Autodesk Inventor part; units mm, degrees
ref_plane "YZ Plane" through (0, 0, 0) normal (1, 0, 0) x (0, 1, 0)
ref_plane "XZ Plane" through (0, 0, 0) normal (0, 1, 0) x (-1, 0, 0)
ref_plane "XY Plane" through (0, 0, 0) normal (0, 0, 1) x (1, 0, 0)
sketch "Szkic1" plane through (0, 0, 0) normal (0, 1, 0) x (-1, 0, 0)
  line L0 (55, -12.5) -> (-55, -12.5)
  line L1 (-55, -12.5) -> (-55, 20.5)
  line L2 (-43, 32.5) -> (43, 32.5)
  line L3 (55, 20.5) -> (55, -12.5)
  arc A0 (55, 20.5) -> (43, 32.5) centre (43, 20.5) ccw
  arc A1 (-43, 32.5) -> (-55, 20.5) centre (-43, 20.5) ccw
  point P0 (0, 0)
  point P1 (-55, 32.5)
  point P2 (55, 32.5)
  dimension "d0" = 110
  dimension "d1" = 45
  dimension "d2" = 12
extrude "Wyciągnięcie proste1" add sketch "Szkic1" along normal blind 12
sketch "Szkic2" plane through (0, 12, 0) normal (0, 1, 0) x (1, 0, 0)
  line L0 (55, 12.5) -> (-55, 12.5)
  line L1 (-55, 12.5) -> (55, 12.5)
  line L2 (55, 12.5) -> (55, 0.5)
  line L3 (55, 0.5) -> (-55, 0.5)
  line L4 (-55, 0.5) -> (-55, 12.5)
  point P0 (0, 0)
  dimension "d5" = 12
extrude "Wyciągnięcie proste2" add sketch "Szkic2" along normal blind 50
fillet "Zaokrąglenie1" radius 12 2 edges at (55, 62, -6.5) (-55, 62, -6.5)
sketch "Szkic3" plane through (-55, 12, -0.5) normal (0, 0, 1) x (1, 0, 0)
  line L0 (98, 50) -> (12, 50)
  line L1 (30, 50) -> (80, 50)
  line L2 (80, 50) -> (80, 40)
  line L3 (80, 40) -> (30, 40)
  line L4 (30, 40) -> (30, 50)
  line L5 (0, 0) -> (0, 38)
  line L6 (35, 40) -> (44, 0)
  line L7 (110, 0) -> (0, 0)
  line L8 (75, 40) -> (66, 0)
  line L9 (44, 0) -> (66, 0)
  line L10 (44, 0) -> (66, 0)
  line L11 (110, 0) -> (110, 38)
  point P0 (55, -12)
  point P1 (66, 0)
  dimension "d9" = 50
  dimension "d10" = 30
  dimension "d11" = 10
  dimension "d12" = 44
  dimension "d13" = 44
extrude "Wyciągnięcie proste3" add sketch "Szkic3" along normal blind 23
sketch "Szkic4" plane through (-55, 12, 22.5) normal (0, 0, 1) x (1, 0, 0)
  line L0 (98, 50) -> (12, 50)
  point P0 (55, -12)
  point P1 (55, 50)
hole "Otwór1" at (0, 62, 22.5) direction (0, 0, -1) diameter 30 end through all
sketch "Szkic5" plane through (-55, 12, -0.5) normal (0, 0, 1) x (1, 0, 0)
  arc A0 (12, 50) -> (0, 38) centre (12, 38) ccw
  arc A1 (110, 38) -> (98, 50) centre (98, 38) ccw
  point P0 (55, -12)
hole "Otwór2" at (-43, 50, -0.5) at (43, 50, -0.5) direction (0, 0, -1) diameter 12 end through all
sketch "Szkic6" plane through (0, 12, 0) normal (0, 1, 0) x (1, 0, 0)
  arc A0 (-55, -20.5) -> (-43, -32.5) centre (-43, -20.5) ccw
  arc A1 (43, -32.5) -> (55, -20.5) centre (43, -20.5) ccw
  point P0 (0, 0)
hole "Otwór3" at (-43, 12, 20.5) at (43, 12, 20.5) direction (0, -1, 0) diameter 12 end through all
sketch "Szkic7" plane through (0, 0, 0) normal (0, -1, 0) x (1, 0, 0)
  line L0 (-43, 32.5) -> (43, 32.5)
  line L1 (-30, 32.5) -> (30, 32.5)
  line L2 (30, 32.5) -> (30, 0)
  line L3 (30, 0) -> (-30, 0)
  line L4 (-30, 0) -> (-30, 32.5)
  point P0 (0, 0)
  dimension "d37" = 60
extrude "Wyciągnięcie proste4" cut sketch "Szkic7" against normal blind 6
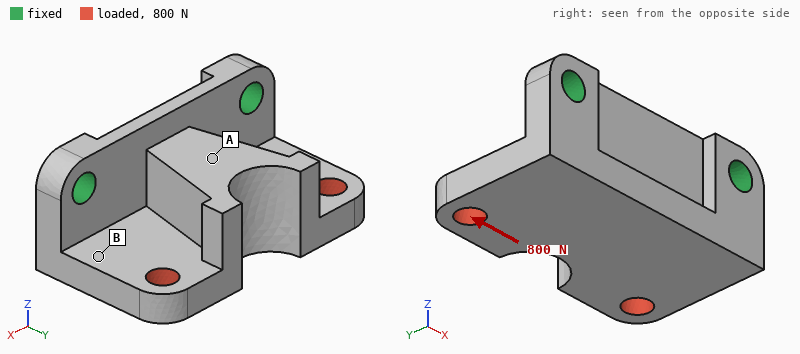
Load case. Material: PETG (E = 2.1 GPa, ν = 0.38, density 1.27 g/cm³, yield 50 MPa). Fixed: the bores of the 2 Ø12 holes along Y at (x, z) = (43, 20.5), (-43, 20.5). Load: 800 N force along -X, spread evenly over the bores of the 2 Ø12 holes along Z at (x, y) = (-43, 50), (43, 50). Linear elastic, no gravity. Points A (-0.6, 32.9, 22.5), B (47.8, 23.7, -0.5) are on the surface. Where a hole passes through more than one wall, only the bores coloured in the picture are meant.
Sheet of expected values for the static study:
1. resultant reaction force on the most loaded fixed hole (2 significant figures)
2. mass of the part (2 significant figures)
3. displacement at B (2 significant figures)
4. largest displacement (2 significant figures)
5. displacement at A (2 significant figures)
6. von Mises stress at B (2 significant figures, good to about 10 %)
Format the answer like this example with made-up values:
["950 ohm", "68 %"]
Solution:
["610 N", "170 g", "0.15 mm", "0.27 mm", "0.11 mm", "2.8 MPa"]
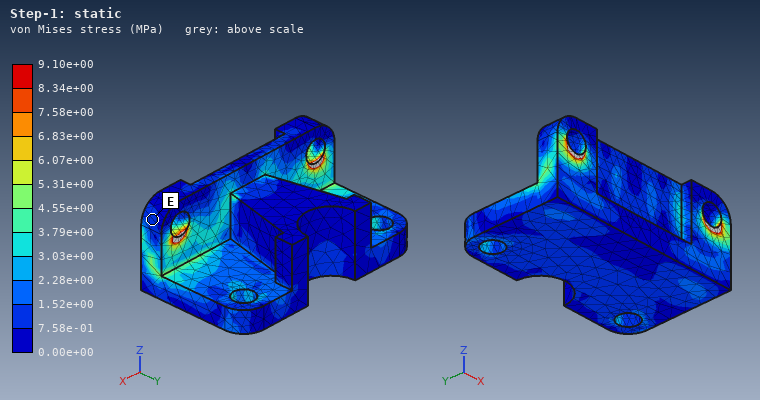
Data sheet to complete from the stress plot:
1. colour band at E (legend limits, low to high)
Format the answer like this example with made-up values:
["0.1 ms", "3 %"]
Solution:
["7.58e-01 to 1.52e+00 MPa"]
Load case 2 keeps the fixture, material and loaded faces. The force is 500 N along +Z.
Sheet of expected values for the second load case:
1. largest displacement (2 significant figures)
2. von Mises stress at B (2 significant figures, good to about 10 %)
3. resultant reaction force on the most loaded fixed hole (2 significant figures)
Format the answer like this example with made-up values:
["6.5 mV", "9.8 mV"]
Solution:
["1.5 mm", "3.5 MPa", "290 N"]
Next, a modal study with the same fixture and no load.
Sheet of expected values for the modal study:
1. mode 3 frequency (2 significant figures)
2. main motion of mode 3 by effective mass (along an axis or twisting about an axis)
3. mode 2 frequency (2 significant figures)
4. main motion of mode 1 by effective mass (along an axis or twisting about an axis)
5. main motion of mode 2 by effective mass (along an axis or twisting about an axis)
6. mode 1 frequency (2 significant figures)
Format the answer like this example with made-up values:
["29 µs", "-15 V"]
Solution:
["1100 Hz", "along Y", "1000 Hz", "along Z", "along X", "410 Hz"]
